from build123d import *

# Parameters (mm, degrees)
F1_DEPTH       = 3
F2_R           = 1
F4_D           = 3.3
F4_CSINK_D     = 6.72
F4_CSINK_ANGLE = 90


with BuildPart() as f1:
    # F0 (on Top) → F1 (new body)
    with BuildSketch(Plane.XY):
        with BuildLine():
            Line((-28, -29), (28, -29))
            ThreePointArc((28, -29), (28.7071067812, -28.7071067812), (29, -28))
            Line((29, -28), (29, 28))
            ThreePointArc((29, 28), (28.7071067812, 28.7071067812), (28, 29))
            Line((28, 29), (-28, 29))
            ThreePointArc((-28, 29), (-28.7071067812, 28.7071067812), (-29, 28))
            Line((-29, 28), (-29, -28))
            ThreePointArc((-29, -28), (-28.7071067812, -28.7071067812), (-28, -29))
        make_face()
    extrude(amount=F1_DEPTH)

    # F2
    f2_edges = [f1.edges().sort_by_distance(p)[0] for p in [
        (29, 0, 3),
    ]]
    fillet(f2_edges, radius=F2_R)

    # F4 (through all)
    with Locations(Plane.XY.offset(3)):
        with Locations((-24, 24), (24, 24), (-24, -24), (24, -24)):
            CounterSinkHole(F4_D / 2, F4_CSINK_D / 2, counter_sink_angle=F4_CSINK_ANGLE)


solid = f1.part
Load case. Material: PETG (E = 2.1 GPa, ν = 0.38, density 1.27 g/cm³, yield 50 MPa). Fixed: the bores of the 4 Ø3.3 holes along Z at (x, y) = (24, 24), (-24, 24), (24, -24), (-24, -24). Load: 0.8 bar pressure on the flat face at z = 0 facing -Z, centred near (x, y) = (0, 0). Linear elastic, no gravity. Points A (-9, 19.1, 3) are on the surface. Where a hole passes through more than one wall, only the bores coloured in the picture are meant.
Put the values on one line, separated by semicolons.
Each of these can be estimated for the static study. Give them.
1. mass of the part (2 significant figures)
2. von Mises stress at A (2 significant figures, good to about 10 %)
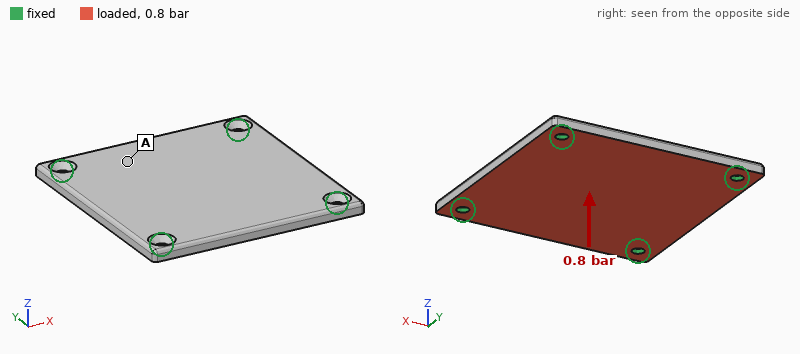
13 g; 6.4 MPa
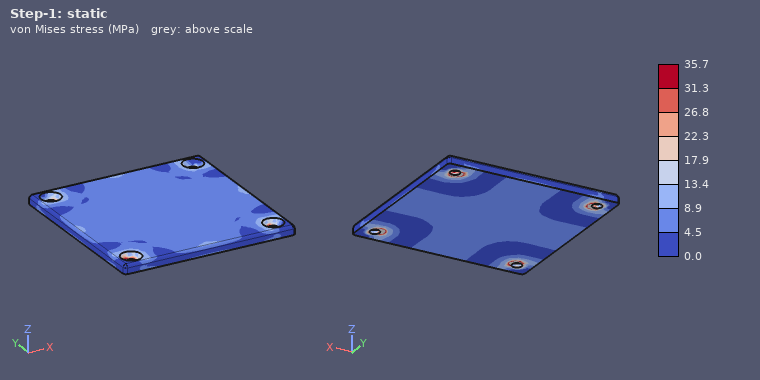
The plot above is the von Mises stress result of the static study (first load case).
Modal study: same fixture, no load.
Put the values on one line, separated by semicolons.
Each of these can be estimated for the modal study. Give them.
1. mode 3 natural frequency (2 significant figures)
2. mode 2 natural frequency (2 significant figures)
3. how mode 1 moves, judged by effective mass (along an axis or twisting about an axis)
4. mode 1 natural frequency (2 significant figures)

1700 Hz; 1700 Hz; along Z; 1000 Hz
